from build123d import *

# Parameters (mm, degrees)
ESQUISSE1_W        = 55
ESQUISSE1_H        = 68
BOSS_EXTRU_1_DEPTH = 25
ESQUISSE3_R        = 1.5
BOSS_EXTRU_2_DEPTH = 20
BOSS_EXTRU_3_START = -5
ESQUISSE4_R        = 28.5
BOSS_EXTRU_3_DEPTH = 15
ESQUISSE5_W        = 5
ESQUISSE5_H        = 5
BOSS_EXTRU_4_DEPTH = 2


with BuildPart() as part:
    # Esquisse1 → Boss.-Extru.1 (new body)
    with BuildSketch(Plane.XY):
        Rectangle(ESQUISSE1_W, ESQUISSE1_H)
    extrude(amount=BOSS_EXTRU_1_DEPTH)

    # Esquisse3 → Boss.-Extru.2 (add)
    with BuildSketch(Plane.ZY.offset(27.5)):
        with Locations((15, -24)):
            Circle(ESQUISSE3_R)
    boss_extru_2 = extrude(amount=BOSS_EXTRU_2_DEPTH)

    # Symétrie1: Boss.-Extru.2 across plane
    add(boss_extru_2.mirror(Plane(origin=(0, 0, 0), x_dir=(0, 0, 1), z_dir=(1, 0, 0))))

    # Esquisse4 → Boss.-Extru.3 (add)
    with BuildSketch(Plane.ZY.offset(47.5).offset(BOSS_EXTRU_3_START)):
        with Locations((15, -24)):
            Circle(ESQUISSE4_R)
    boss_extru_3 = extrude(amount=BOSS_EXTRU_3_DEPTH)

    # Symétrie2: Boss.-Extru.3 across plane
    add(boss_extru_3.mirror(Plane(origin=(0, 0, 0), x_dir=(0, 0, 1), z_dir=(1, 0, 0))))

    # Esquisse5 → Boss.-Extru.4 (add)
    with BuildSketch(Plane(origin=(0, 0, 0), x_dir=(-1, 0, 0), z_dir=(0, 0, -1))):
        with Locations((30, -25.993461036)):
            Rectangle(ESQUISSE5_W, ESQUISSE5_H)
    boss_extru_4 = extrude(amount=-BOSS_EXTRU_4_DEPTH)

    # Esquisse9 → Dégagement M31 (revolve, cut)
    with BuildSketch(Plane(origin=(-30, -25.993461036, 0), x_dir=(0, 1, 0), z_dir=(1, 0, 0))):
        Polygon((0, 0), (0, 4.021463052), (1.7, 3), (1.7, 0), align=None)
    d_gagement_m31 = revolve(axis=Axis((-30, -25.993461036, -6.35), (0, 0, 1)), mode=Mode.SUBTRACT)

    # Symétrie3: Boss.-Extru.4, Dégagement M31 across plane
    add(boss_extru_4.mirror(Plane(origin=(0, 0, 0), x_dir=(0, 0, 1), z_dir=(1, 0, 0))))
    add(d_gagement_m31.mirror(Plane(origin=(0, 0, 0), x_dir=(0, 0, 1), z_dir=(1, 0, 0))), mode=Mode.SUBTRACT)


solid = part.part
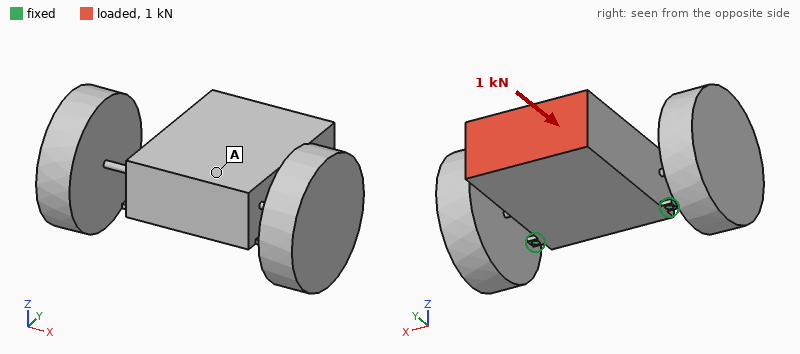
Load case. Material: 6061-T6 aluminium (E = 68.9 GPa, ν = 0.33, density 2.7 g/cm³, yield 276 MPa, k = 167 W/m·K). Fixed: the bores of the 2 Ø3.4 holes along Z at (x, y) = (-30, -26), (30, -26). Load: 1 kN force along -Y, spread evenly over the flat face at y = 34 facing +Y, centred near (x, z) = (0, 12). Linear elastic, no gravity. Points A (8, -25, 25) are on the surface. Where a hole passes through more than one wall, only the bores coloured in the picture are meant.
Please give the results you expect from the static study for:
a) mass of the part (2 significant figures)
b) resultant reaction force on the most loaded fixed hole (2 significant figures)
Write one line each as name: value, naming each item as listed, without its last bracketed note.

mass of the part: 460 g
resultant reaction force on the most loaded fixed hole: 500 N
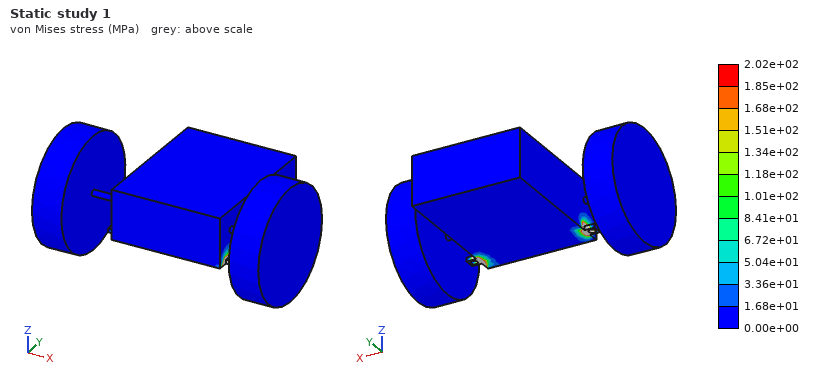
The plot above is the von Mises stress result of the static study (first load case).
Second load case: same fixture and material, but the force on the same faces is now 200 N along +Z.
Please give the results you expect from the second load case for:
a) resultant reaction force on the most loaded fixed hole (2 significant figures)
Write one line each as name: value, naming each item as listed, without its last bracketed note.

resultant reaction force on the most loaded fixed hole: 110 N
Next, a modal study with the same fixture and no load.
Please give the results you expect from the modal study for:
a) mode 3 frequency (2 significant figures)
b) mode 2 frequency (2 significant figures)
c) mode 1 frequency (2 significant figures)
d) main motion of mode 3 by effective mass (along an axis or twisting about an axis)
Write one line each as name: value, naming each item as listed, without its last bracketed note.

mode 3 frequency: 94 Hz
mode 2 frequency: 89 Hz
mode 1 frequency: 85 Hz
main motion of mode 3 by effective mass: along Y
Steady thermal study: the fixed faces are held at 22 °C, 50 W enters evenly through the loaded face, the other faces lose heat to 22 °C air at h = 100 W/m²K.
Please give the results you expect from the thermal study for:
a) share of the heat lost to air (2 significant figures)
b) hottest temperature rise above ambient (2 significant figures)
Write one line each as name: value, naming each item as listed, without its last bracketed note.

share of the heat lost to air: 59 %
hottest temperature rise above ambient: 29 K
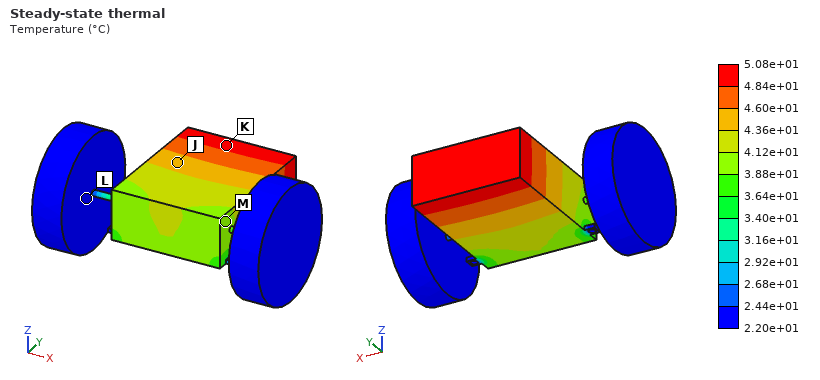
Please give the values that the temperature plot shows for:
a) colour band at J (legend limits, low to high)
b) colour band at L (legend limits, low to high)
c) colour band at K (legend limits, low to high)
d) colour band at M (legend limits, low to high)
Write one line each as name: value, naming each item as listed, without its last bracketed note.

colour band at J: 4.36e+01 to 4.60e+01 °C
colour band at L: 2.20e+01 to 2.44e+01 °C
colour band at K: 4.84e+01 to 5.08e+01 °C
colour band at M: 3.88e+01 to 4.12e+01 °C
